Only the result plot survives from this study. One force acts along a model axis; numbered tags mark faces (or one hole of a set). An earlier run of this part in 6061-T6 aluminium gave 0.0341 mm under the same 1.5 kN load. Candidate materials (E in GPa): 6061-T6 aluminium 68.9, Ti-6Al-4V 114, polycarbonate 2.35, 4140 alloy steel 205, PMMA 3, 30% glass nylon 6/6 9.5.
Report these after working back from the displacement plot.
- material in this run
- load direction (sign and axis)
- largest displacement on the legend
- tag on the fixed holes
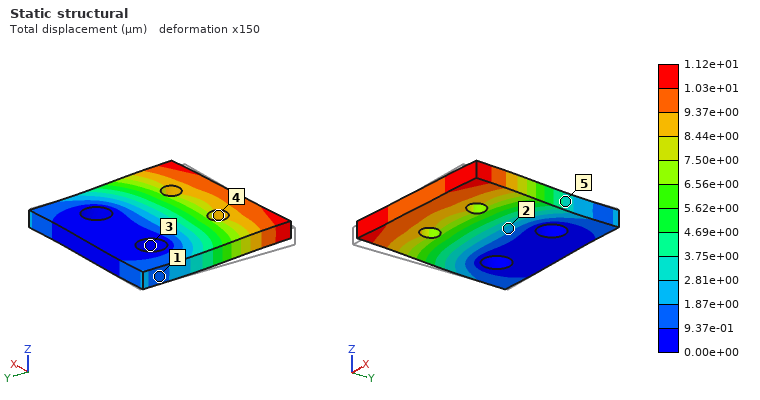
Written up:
4140 alloy steel
+X
1.12e+01 µm
3
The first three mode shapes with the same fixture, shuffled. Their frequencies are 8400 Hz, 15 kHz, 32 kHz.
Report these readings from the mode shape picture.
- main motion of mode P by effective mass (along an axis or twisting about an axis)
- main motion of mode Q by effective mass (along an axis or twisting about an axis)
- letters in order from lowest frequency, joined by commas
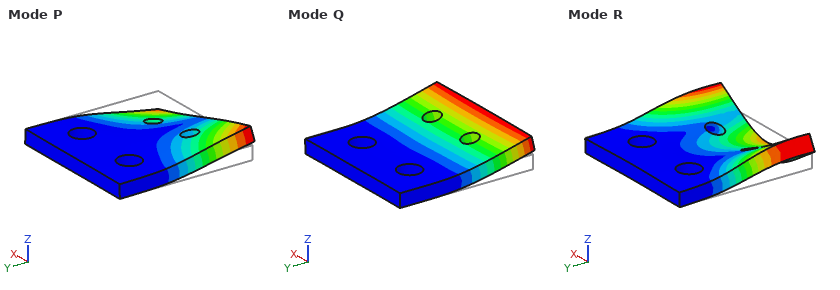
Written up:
twisting about Y
along Z
Q, P, R
